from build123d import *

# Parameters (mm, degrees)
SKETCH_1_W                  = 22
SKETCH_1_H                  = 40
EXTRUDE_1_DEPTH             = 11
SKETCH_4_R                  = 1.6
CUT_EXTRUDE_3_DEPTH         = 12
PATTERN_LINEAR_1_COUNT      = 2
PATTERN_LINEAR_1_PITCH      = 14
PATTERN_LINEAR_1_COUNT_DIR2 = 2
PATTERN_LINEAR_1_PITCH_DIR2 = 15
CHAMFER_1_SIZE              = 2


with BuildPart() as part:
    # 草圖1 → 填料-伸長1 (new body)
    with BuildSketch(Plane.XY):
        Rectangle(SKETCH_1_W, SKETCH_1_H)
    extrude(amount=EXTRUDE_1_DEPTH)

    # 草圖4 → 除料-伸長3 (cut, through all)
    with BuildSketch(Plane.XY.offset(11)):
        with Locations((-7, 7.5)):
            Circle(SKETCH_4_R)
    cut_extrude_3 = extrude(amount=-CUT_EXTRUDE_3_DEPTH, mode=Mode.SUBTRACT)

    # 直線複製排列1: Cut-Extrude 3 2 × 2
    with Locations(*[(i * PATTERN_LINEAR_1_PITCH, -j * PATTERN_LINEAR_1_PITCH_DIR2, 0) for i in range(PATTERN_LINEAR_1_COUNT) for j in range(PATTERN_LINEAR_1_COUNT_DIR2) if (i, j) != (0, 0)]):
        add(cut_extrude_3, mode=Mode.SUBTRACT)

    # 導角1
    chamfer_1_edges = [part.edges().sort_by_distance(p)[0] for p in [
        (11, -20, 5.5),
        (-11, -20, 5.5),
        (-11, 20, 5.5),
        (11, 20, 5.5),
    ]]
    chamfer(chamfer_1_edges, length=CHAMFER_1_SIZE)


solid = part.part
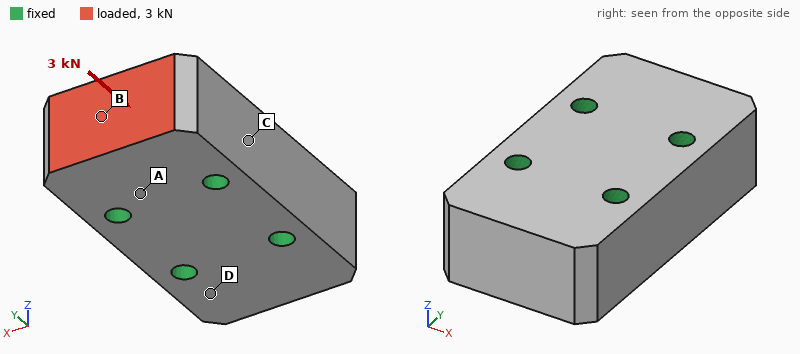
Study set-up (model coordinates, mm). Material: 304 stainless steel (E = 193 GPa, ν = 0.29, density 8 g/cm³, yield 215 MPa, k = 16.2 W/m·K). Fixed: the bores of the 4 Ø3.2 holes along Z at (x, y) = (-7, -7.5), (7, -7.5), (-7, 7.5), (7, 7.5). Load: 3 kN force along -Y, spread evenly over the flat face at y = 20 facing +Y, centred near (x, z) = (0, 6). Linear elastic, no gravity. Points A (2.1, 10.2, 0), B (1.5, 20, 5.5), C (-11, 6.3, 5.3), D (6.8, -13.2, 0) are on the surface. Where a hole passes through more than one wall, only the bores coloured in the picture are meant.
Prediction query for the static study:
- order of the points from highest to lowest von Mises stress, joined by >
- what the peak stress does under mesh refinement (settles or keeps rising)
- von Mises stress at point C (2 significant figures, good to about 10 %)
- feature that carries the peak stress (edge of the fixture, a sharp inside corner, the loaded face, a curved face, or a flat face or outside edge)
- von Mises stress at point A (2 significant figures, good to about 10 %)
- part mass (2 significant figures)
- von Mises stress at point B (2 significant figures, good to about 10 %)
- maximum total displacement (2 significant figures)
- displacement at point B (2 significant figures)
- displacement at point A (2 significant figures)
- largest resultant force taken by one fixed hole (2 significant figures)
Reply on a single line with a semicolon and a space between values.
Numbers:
B > A > C > D; keeps rising; 5.7 MPa; edge of the fixture; 9.0 MPa; 74 g; 13 MPa; 1.0 µm; 0.99 µm; 0.37 µm; 1.4 kN
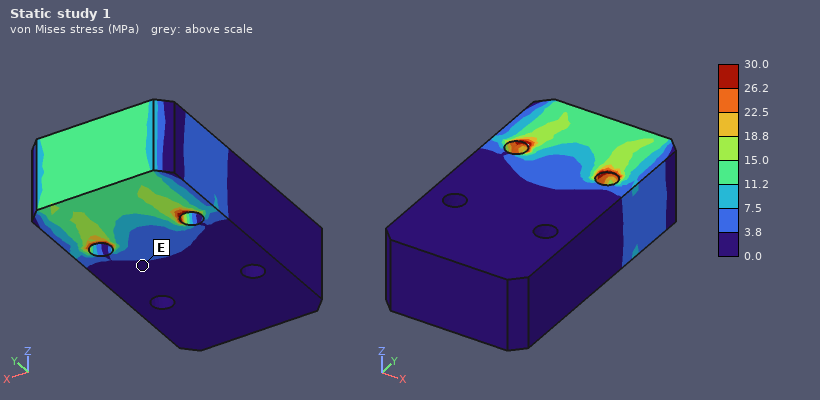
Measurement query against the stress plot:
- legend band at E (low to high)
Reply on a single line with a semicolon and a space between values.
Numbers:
0.0 to 3.8 MPa
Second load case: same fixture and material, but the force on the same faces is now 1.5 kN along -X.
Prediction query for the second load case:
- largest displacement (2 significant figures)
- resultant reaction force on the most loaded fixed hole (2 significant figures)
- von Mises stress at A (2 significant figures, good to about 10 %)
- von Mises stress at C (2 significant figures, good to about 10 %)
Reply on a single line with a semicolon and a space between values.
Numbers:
1.9 µm; 1.3 kN; 12 MPa; 11 MPa
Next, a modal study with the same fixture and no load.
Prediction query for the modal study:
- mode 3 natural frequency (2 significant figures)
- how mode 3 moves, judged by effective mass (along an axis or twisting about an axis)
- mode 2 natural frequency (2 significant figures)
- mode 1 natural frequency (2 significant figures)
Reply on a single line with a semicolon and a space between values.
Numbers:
51 kHz; twisting about Z; 39 kHz; 38 kHz
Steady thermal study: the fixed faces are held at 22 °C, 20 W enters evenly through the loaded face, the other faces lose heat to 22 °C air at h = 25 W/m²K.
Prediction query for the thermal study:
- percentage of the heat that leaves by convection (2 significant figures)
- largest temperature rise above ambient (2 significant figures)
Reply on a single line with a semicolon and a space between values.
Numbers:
3.3 %; 68 K
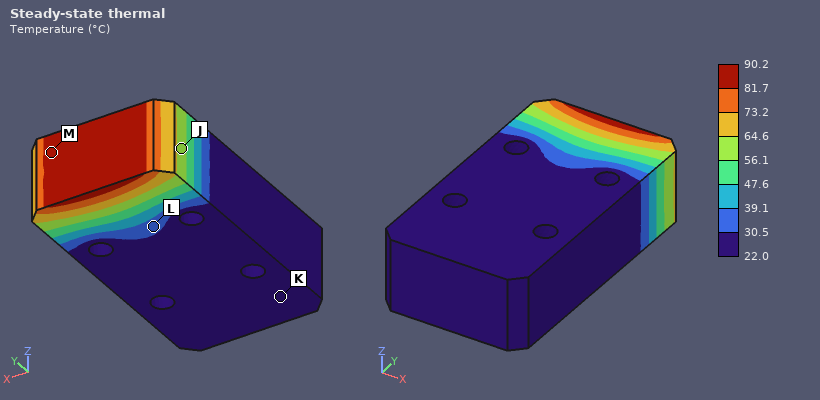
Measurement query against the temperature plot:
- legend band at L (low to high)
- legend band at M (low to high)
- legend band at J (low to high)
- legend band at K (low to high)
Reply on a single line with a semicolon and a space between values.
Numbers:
30.5 to 39.1 °C; 81.7 to 90.2 °C; 56.1 to 64.6 °C; 22.0 to 30.5 °C
